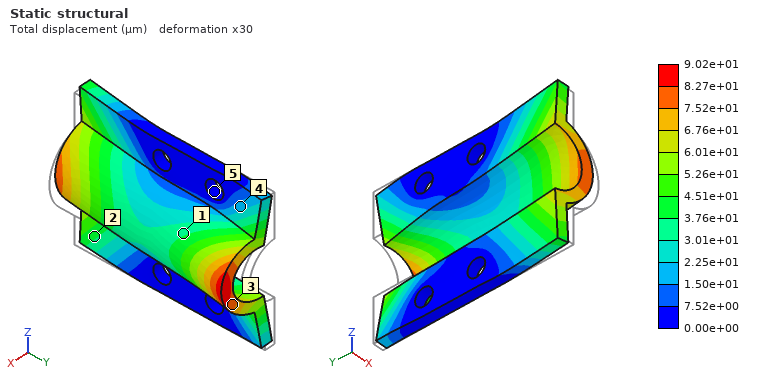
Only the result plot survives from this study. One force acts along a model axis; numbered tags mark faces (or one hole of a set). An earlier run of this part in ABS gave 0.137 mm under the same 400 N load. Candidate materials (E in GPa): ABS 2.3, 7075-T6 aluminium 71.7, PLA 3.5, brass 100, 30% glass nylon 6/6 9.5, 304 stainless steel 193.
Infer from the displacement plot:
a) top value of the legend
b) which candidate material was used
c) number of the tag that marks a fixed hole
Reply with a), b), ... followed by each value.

a) 9.02e+01 µm
b) PLA
c) 5
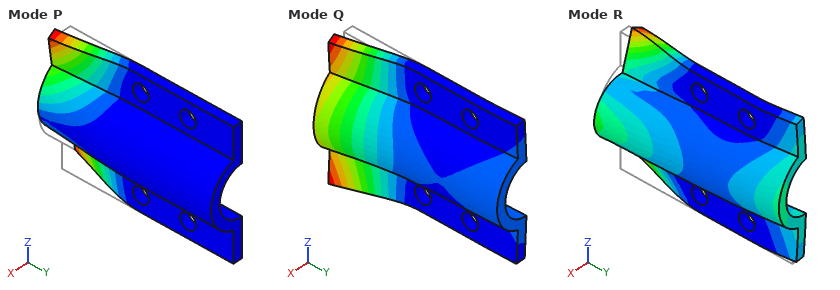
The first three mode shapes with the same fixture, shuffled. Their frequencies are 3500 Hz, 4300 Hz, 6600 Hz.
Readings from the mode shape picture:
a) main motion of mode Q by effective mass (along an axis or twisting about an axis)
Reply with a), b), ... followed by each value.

a) along X
